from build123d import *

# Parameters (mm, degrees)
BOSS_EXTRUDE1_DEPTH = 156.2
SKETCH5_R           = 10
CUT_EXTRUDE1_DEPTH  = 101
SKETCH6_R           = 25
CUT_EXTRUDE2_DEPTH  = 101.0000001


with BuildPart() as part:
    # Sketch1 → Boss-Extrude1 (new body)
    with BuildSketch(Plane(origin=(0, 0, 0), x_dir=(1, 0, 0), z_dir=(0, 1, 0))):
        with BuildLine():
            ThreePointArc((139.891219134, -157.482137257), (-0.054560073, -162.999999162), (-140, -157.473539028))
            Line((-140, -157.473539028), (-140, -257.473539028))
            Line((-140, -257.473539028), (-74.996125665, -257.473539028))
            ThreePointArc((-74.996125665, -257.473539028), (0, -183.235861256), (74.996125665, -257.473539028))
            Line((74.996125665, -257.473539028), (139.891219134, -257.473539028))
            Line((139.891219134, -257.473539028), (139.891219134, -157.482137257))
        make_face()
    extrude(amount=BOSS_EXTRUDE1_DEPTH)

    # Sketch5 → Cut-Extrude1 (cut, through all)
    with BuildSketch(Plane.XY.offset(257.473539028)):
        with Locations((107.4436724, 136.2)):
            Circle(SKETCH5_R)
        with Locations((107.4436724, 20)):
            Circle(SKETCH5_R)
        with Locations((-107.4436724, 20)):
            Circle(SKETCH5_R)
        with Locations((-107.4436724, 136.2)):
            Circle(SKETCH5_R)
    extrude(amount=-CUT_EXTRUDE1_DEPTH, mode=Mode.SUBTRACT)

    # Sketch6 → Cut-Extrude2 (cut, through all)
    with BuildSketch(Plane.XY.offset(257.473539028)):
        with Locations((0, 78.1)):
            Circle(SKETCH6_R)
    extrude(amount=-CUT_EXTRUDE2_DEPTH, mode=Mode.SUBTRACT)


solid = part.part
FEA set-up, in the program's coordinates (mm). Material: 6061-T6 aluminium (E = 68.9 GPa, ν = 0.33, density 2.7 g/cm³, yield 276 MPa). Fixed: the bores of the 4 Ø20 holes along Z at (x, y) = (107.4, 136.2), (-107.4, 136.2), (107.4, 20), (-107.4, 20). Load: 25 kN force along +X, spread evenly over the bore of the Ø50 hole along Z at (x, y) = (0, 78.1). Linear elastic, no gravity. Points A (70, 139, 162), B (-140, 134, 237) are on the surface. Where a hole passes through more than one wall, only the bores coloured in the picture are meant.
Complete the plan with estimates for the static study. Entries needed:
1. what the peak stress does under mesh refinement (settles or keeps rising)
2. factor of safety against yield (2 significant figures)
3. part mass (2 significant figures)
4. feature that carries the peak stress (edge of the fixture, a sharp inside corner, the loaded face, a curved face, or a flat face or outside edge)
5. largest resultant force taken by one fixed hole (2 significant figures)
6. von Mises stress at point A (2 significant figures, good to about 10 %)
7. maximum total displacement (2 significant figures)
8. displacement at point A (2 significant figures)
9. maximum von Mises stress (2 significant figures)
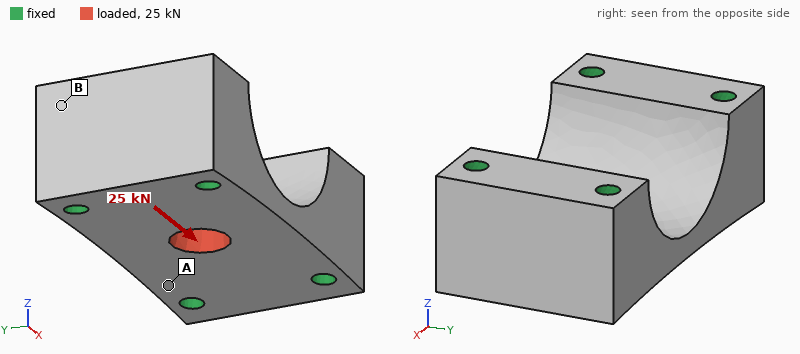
settles
19
7.2 kg
the loaded face
6.5 kN
2.5 MPa
7.4 µm
1.4 µm
15 MPa
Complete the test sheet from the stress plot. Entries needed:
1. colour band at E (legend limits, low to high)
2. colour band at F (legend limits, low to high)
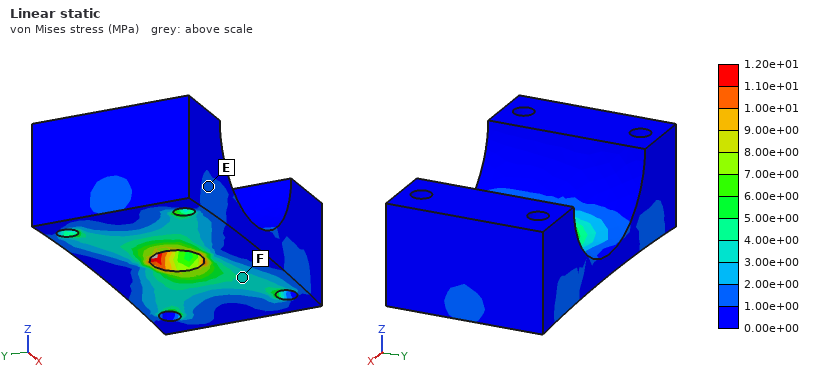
1.00e+00 to 2.00e+00 MPa
3.00e+00 to 4.00e+00 MPa
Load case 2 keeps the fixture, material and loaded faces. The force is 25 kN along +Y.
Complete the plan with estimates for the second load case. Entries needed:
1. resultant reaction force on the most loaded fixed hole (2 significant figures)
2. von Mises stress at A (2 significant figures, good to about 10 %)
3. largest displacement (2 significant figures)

9.4 kN
2.9 MPa
12 µm
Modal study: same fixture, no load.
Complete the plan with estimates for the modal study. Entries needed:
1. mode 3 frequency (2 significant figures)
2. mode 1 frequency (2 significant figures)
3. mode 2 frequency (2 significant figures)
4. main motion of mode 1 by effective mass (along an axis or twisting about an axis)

8600 Hz
6700 Hz
7700 Hz
along Z
